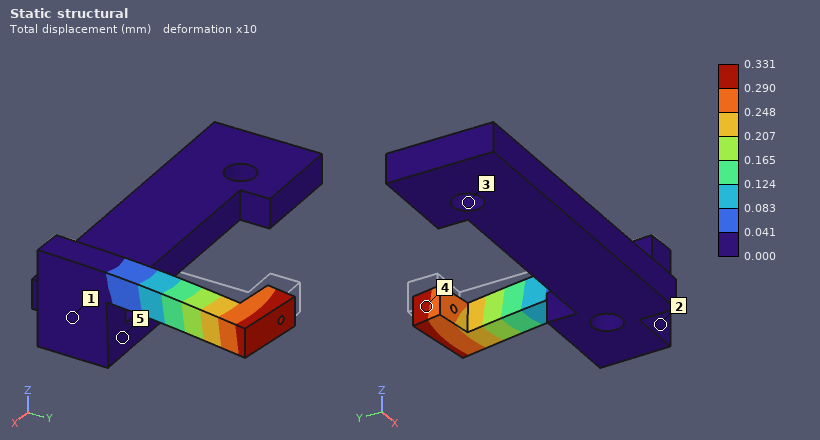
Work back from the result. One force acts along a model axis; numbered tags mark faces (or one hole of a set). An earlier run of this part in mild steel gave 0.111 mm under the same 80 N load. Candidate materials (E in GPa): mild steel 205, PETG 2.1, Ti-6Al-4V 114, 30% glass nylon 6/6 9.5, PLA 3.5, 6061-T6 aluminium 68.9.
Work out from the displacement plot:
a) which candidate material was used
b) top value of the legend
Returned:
6061-T6 aluminium
0.331 mm
